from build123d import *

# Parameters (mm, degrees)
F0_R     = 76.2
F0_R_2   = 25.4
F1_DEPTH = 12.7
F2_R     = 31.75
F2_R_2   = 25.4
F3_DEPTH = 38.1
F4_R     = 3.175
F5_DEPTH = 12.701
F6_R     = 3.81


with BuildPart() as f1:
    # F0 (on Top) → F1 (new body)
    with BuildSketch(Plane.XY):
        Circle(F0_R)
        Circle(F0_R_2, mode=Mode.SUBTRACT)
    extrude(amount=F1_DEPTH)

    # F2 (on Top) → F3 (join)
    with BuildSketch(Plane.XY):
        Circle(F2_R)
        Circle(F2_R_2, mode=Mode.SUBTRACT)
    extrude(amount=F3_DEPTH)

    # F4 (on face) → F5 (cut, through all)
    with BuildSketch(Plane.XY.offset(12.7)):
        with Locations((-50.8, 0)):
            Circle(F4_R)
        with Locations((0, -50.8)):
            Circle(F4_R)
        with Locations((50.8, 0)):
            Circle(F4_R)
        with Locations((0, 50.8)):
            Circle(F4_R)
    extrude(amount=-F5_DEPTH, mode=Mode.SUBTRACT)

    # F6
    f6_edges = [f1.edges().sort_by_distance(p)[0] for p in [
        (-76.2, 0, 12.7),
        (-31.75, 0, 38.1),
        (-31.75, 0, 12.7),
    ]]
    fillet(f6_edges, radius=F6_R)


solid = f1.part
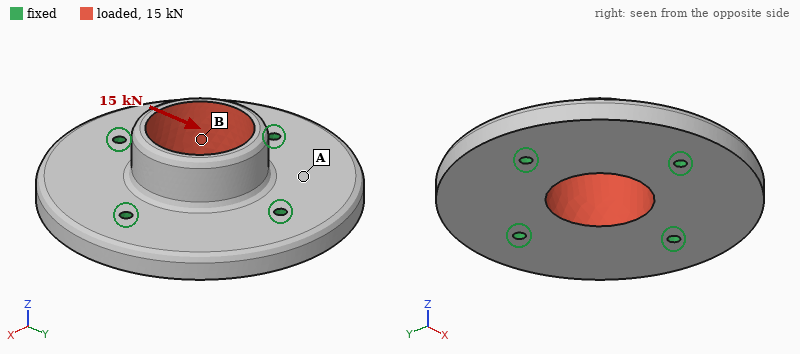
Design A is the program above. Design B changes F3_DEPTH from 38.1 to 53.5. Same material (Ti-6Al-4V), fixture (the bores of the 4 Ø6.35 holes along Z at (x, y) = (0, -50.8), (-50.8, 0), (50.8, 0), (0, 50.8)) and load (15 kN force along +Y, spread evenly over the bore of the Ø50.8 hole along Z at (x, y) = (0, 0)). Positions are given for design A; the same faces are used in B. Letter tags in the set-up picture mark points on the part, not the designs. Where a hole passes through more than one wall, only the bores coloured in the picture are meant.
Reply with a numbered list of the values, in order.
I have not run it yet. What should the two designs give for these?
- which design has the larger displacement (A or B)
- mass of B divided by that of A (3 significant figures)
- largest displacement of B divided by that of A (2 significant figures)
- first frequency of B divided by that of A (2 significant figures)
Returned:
1. B
2. 1.08
3. 1.8
4. 1.0
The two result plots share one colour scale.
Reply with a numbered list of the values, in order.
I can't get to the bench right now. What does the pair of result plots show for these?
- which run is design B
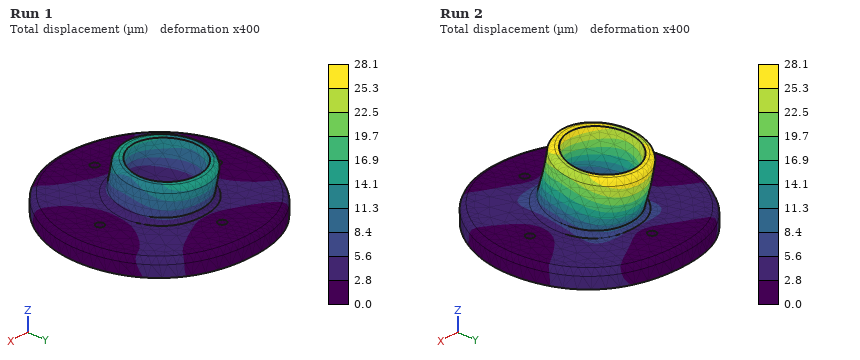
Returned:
1. Run 2
